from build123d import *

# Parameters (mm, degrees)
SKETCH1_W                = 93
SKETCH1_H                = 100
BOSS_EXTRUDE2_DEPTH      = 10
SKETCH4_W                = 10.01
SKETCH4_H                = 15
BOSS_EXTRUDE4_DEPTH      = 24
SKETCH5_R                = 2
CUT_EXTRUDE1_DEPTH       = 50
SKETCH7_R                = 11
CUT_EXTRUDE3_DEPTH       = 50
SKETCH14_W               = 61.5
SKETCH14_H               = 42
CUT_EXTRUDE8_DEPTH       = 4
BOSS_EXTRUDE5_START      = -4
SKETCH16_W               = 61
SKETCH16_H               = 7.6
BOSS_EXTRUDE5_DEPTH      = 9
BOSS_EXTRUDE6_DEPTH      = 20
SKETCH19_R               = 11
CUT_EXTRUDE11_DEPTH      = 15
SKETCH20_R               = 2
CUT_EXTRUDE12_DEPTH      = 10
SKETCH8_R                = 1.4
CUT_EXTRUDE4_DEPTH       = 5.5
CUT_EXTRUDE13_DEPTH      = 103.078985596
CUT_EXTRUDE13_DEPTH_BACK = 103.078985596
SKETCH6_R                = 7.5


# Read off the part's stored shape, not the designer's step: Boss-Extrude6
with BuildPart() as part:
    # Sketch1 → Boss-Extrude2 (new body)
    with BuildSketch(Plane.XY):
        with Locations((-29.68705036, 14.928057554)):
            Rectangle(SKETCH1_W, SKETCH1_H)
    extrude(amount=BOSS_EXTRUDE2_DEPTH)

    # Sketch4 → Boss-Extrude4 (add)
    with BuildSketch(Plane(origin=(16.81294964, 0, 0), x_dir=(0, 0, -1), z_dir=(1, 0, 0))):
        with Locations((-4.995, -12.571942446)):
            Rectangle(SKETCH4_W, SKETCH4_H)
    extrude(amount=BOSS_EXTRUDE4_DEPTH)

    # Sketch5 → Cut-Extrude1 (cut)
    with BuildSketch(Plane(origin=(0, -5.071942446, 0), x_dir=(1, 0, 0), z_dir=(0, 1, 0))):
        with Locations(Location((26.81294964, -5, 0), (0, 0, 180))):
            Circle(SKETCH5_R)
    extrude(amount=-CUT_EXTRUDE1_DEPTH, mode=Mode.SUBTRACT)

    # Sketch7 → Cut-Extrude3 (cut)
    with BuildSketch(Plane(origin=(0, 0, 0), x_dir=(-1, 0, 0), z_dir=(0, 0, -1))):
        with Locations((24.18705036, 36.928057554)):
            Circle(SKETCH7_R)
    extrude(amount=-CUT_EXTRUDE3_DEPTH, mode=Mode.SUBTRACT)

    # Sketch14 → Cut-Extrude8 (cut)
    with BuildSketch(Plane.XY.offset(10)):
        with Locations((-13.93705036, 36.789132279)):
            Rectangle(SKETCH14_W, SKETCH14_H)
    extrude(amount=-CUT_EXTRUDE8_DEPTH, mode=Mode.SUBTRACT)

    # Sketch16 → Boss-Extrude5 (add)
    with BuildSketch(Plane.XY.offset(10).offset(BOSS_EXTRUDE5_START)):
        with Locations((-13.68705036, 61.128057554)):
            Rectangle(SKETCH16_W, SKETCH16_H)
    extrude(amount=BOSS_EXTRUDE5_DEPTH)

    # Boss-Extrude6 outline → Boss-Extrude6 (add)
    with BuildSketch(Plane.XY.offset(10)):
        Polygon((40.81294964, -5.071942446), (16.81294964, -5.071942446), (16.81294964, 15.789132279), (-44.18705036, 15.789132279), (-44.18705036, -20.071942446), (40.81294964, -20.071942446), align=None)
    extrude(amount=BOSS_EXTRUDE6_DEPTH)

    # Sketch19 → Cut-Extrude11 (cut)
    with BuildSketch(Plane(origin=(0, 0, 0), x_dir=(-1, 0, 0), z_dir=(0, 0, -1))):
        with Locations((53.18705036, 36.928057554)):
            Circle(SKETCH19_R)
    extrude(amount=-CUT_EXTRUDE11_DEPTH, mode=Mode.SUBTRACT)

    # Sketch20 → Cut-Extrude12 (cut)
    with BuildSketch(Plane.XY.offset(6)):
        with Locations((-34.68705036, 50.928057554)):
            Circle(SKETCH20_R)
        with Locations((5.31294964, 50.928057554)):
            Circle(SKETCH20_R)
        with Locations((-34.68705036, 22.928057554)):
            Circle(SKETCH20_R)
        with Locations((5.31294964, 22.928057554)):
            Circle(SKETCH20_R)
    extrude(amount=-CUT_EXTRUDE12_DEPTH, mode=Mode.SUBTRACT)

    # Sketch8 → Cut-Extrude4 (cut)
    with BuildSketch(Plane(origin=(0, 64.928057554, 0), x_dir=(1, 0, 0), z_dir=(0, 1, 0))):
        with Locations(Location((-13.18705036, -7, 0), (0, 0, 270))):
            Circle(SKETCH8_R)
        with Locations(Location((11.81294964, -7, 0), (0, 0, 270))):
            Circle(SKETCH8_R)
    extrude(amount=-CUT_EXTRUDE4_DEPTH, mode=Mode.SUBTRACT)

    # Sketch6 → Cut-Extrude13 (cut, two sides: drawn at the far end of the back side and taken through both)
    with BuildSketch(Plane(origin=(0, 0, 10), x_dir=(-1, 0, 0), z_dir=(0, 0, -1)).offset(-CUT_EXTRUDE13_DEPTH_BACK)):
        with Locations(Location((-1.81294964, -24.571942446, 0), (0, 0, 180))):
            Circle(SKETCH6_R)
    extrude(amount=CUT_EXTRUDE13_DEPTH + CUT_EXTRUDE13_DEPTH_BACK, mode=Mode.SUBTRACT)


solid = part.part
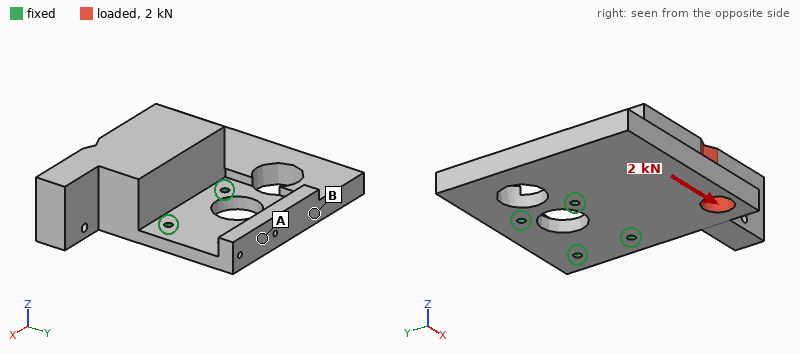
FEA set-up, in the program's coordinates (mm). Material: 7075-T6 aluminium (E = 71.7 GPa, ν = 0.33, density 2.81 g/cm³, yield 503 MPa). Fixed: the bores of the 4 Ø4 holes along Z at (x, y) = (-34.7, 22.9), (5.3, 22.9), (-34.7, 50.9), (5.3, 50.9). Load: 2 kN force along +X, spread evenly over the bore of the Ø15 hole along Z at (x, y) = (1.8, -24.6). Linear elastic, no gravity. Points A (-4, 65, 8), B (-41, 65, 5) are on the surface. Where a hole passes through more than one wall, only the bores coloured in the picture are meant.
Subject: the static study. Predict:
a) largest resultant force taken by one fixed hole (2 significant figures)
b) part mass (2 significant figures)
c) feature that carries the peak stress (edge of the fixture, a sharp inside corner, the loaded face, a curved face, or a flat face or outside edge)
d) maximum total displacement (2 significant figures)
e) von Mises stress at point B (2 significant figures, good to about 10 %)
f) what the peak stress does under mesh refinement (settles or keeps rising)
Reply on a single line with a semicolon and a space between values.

2.0 kN; 370 g; edge of the fixture; 21 µm; 5.3 MPa; keeps rising
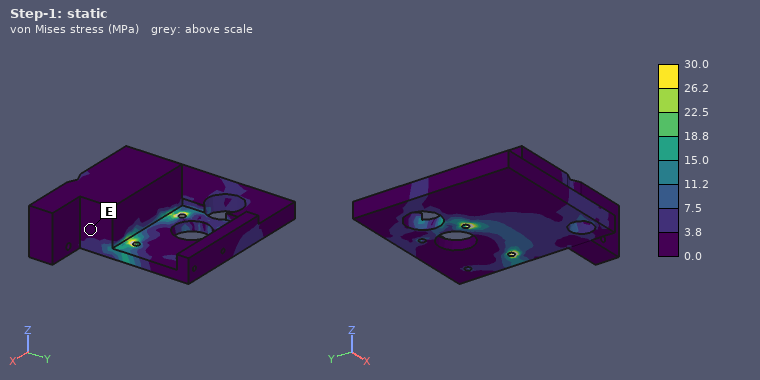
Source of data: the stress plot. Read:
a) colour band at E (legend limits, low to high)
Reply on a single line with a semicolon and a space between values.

0.0 to 3.8 MPa
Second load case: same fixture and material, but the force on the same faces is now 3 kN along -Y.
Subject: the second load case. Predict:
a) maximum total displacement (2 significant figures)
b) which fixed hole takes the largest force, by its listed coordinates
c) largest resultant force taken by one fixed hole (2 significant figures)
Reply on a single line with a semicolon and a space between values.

0.13 mm; (5.3, 22.9); 2.2 kN
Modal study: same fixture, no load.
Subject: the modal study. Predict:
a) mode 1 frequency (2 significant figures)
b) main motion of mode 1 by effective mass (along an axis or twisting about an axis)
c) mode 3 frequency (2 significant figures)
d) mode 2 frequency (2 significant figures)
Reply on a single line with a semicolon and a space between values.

940 Hz; along Z; 4100 Hz; 2700 Hz
